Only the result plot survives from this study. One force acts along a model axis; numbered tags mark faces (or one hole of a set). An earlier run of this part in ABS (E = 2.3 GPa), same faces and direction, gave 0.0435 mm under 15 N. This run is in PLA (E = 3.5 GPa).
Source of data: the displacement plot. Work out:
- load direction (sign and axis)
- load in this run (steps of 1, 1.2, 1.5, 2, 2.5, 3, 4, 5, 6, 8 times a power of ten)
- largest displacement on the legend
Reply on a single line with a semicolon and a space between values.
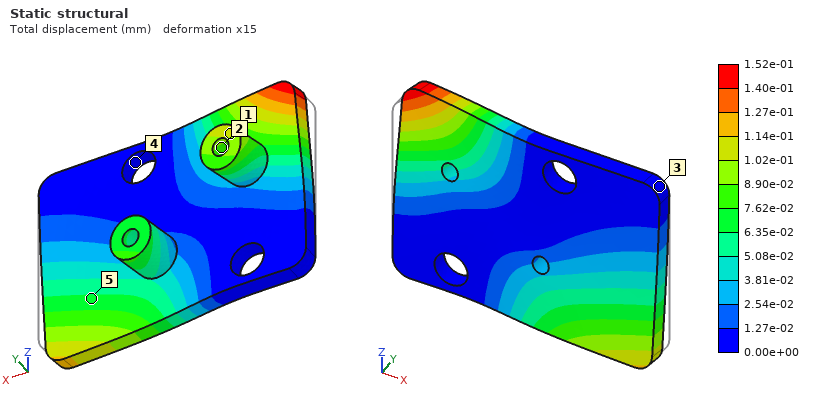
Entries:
-Z; 80 N; 1.52e-01 mm
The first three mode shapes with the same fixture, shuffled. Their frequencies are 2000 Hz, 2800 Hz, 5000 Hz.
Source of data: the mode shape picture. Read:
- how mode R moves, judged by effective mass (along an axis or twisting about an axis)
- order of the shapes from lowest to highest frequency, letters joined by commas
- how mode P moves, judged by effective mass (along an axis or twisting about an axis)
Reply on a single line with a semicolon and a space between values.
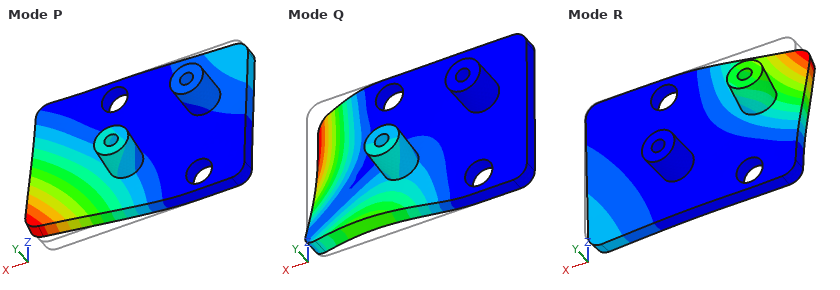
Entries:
along Y; P, R, Q; along Y
